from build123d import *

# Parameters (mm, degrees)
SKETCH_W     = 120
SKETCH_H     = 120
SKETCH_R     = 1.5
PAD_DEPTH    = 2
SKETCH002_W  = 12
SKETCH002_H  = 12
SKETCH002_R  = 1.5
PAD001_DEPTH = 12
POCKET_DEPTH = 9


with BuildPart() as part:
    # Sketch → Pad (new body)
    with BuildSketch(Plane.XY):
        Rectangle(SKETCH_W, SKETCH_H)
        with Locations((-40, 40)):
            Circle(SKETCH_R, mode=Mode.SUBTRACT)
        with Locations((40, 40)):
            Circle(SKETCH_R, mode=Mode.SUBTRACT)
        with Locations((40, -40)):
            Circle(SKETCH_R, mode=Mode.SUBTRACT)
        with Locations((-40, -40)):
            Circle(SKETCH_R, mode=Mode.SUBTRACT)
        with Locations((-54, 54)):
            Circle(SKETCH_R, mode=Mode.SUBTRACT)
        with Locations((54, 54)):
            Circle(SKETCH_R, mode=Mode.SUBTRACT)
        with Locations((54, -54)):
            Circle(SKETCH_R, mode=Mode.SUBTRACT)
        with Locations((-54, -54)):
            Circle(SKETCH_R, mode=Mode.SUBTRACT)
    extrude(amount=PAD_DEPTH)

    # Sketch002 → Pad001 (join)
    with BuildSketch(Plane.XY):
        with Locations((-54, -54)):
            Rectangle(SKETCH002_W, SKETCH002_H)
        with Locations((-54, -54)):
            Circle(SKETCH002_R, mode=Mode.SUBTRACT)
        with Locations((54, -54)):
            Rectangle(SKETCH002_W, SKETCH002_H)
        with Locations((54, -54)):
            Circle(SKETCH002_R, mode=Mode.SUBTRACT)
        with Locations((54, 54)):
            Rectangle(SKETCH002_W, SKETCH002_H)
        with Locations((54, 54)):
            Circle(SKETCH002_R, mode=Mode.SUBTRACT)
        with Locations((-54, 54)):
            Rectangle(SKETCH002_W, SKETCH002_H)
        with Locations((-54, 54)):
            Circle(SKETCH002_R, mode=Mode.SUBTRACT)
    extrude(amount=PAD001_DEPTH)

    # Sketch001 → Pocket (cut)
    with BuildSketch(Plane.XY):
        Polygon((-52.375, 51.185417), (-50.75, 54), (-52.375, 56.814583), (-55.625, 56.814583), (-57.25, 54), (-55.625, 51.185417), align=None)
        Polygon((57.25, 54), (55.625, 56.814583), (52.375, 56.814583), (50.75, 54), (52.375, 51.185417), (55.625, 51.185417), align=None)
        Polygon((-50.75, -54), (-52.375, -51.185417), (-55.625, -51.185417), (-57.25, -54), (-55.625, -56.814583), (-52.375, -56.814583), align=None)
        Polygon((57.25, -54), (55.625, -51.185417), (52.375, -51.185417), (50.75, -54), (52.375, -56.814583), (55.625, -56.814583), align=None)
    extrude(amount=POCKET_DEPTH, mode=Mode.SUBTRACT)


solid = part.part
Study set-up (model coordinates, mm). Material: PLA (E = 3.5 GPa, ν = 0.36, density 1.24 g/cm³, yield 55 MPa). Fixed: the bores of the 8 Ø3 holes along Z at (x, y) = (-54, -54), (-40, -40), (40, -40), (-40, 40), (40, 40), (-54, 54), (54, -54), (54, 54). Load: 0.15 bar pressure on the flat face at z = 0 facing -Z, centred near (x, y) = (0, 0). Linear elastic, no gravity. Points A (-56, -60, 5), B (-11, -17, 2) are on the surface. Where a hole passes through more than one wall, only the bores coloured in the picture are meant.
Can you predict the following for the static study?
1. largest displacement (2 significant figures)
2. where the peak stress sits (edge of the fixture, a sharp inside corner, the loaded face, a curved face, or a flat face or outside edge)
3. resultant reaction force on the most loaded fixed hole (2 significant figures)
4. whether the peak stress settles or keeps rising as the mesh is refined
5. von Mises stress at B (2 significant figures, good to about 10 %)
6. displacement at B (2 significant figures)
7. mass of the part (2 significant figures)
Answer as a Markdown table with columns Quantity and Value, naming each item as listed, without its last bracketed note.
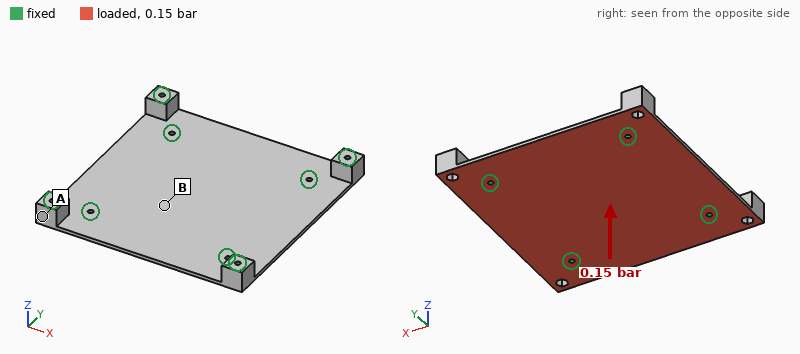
| Quantity | Value |
|---|---|
| largest displacement | 1.6 mm |
| where the peak stress sits | edge of the fixture |
| resultant reaction force on the most loaded fixed hole | 60 N |
| whether the peak stress settles or keeps rising as the mesh is refined | keeps rising |
| von Mises stress at B | 5.7 MPa |
| displacement at B | 1.3 mm |
| mass of the part | 41 g |
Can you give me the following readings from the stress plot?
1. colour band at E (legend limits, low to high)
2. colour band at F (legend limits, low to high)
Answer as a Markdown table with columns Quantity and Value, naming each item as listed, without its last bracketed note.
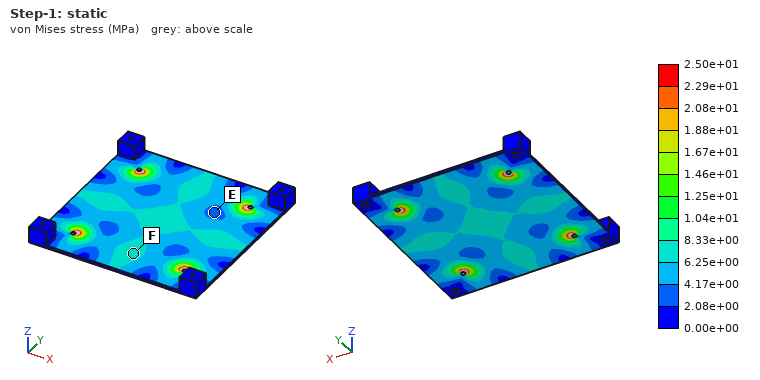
| Quantity | Value |
|---|---|
| colour band at E | 2.08e+00 to 4.17e+00 MPa |
| colour band at F | 6.25e+00 to 8.33e+00 MPa |
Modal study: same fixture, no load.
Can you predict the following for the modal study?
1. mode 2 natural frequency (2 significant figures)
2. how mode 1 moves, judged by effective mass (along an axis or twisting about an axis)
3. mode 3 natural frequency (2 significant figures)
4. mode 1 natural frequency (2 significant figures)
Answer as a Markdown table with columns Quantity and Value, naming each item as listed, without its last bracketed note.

| Quantity | Value |
|---|---|
| mode 2 natural frequency | 520 Hz |
| how mode 1 moves, judged by effective mass | along Z |
| mode 3 natural frequency | 530 Hz |
| mode 1 natural frequency | 390 Hz |
